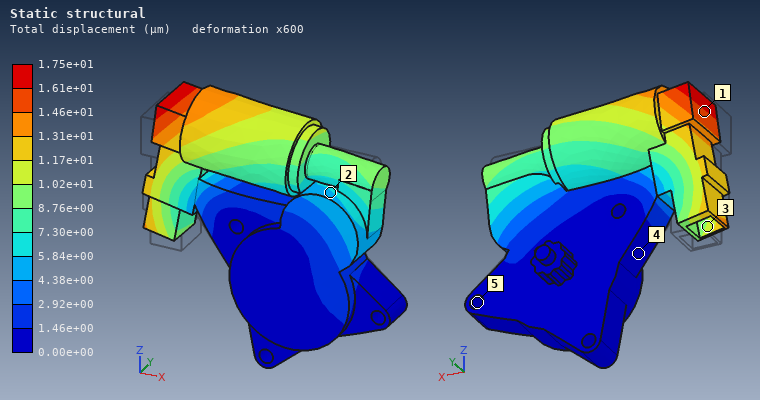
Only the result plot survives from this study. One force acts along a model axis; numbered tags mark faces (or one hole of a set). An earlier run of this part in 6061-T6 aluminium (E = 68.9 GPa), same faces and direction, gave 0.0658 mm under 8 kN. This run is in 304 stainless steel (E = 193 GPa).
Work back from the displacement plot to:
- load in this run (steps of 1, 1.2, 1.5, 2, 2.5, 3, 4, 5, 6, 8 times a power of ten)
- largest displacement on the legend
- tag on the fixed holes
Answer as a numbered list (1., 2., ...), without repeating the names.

1. 6 kN
2. 1.75e+01 µm
3. 5
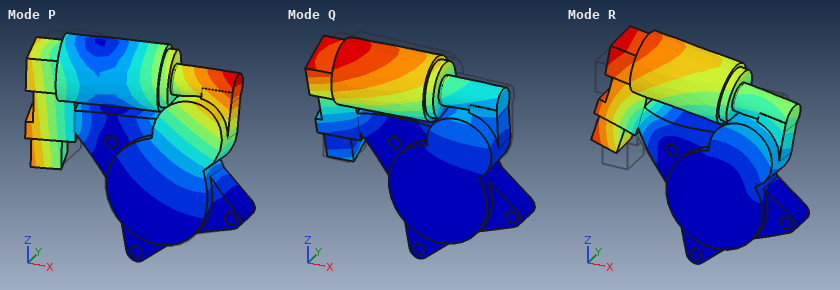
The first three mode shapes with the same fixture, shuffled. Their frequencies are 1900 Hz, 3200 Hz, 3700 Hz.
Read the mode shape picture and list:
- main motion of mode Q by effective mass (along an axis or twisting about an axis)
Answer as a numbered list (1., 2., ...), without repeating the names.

1. along Y
